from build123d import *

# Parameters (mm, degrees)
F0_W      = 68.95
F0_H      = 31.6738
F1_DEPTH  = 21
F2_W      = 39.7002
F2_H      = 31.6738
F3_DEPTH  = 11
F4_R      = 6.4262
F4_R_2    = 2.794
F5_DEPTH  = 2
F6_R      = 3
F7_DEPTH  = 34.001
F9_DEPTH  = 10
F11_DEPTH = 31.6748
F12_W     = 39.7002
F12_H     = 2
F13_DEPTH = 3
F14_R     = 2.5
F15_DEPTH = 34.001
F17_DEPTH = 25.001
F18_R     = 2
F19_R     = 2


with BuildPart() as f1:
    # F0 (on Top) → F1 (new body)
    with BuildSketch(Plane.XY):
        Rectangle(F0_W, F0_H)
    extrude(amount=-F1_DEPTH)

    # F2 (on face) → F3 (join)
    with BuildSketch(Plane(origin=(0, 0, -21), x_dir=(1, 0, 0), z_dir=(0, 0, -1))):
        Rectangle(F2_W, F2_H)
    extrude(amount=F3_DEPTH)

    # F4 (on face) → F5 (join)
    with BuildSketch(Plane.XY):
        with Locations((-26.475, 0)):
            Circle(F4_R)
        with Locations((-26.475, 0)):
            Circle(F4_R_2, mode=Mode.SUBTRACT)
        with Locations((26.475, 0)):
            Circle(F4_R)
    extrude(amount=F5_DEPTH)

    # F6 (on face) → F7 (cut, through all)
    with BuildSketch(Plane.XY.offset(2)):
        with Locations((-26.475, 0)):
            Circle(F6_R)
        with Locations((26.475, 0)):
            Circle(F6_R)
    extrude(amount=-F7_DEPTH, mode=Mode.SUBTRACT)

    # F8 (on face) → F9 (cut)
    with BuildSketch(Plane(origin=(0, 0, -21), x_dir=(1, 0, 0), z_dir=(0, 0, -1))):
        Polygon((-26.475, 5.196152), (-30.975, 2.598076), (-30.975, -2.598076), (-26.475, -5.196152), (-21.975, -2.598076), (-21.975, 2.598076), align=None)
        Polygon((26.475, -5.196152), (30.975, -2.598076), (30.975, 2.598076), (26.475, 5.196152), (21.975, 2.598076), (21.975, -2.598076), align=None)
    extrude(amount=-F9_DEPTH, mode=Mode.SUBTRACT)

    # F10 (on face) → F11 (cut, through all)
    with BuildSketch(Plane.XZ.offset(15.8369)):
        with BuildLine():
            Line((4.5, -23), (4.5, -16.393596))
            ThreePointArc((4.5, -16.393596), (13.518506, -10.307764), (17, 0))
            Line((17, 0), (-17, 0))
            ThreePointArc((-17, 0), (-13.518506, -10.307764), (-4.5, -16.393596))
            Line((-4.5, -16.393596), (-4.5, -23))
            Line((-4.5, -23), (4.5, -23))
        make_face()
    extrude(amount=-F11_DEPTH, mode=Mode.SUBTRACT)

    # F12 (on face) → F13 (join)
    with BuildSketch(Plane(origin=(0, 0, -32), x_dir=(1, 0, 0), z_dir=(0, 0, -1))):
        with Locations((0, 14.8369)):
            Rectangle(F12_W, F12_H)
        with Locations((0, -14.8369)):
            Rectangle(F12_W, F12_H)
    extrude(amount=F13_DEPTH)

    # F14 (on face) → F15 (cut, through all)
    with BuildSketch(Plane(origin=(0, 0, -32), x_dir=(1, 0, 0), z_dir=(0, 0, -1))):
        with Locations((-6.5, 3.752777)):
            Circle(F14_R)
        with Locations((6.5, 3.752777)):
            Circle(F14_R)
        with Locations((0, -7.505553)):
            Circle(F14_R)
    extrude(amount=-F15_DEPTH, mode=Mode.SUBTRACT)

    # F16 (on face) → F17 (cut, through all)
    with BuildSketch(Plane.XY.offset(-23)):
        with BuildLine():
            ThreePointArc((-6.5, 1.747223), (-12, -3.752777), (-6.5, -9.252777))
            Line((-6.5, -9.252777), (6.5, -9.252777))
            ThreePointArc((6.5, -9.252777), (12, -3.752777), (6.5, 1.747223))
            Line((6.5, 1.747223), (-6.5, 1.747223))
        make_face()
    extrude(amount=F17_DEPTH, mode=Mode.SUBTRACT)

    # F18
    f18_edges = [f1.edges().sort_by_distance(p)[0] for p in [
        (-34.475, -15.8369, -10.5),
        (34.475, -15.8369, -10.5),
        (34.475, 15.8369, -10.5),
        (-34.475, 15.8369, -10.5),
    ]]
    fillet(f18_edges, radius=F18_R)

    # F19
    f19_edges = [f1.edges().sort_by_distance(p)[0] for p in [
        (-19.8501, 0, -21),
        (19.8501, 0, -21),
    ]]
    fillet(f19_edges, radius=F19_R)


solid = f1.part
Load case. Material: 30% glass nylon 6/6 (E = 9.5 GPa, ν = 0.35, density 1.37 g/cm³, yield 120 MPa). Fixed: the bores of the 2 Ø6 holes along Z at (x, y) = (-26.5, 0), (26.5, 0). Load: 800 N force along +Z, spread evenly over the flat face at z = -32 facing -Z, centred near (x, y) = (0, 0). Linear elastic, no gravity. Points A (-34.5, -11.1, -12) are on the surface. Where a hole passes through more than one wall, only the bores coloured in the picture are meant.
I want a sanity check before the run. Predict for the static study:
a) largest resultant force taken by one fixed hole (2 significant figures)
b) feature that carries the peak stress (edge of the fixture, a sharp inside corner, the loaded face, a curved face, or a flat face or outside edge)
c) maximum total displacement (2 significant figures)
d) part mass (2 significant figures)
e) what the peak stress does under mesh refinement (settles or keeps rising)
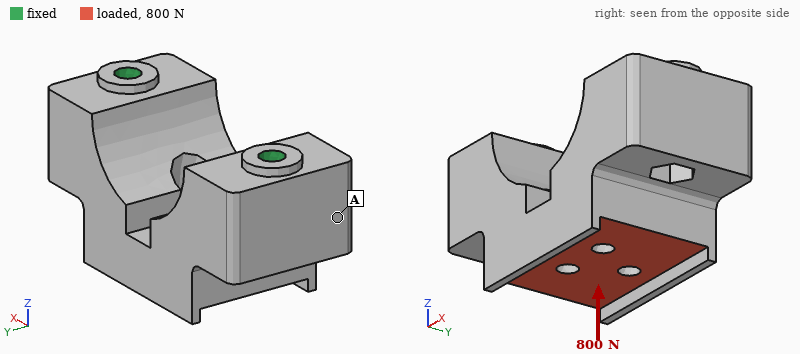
460 N
edge of the fixture
8.7 µm
56 g
keeps rising
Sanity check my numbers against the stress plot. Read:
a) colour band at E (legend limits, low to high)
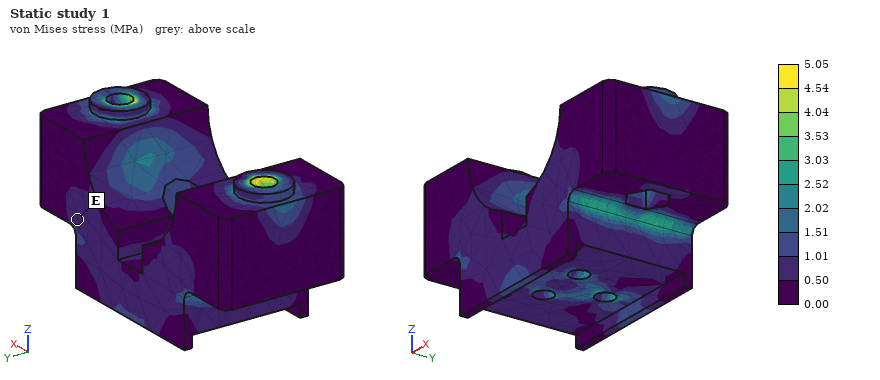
0.50 to 1.01 MPa
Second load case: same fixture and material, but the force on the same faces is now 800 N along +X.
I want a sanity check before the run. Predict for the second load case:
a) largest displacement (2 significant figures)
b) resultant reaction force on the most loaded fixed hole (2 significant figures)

15 µm
530 N
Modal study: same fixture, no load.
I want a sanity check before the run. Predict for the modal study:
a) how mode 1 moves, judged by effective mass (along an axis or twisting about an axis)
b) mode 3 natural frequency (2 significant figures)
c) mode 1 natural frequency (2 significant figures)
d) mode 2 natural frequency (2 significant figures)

along Y
7900 Hz
4000 Hz
7800 Hz
